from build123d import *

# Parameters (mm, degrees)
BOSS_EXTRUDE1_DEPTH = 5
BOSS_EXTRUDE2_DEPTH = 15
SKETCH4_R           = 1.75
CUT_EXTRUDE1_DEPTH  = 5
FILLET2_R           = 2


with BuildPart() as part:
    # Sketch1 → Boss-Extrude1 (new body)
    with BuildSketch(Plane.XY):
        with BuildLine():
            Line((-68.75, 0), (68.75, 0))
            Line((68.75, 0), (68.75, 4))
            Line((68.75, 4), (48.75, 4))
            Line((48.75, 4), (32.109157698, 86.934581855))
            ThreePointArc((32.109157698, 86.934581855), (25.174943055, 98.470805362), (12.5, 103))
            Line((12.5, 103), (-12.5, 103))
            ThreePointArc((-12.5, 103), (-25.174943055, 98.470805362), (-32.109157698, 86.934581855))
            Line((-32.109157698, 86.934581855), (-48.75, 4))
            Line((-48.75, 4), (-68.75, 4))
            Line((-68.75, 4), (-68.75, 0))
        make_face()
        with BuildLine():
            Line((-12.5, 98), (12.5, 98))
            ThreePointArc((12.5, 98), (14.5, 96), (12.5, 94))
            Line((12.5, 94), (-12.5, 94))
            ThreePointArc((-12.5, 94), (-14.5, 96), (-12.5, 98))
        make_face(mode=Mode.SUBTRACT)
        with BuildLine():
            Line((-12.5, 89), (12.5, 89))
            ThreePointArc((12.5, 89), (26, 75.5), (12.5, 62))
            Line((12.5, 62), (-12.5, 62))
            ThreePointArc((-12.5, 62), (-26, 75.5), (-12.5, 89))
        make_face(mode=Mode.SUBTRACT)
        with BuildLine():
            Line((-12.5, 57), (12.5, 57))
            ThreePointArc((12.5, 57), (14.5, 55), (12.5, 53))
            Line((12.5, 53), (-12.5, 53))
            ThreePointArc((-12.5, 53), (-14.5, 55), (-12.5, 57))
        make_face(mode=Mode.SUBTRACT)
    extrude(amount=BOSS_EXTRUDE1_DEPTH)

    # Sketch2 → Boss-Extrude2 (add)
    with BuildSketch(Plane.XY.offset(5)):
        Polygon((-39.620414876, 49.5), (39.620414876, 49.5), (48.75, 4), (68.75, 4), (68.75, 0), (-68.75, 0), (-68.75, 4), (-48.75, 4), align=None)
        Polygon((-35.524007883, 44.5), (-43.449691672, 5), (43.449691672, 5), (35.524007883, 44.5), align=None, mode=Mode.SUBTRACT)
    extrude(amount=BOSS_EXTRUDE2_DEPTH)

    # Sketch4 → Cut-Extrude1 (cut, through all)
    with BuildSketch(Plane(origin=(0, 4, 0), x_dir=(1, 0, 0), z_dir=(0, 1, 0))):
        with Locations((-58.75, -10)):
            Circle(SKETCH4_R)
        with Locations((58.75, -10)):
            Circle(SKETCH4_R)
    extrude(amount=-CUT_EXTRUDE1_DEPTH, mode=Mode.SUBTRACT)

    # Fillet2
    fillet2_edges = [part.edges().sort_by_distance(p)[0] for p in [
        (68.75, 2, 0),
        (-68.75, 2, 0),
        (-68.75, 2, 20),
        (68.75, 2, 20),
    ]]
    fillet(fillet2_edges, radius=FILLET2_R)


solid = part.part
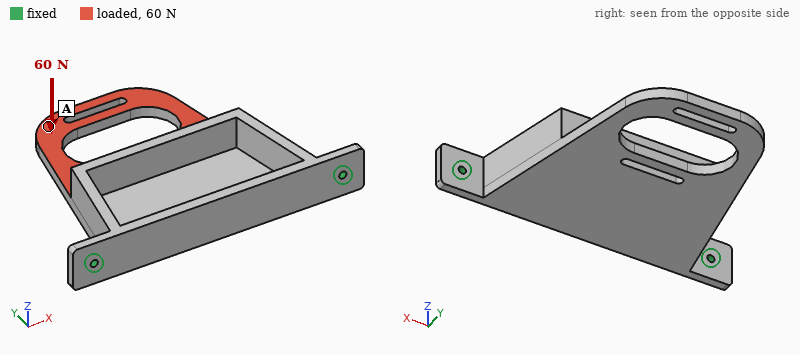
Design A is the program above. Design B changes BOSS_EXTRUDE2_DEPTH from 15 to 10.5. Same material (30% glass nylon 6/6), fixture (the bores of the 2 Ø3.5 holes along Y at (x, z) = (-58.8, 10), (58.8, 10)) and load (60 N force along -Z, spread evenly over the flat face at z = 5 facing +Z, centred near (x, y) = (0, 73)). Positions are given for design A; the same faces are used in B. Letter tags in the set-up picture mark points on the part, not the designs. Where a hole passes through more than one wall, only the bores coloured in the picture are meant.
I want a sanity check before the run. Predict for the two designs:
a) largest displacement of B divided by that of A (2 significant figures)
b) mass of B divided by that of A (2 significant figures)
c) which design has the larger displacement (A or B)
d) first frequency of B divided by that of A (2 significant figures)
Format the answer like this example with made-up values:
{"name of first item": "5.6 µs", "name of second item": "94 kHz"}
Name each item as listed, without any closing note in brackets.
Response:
{"largest displacement of B divided by that of A": "1.4", "mass of B divided by that of A": "0.88", "which design has the larger displacement": "B", "first frequency of B divided by that of A": "0.87"}
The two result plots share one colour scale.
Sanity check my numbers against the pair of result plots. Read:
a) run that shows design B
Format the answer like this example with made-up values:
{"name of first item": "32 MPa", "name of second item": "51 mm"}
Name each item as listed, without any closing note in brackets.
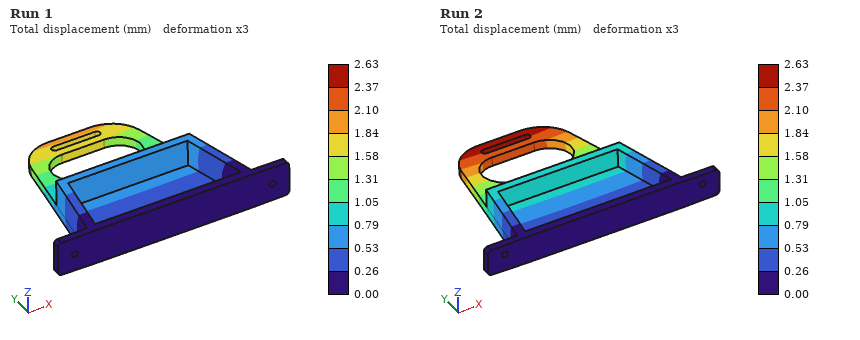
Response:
{"run that shows design B": "Run 2"}
